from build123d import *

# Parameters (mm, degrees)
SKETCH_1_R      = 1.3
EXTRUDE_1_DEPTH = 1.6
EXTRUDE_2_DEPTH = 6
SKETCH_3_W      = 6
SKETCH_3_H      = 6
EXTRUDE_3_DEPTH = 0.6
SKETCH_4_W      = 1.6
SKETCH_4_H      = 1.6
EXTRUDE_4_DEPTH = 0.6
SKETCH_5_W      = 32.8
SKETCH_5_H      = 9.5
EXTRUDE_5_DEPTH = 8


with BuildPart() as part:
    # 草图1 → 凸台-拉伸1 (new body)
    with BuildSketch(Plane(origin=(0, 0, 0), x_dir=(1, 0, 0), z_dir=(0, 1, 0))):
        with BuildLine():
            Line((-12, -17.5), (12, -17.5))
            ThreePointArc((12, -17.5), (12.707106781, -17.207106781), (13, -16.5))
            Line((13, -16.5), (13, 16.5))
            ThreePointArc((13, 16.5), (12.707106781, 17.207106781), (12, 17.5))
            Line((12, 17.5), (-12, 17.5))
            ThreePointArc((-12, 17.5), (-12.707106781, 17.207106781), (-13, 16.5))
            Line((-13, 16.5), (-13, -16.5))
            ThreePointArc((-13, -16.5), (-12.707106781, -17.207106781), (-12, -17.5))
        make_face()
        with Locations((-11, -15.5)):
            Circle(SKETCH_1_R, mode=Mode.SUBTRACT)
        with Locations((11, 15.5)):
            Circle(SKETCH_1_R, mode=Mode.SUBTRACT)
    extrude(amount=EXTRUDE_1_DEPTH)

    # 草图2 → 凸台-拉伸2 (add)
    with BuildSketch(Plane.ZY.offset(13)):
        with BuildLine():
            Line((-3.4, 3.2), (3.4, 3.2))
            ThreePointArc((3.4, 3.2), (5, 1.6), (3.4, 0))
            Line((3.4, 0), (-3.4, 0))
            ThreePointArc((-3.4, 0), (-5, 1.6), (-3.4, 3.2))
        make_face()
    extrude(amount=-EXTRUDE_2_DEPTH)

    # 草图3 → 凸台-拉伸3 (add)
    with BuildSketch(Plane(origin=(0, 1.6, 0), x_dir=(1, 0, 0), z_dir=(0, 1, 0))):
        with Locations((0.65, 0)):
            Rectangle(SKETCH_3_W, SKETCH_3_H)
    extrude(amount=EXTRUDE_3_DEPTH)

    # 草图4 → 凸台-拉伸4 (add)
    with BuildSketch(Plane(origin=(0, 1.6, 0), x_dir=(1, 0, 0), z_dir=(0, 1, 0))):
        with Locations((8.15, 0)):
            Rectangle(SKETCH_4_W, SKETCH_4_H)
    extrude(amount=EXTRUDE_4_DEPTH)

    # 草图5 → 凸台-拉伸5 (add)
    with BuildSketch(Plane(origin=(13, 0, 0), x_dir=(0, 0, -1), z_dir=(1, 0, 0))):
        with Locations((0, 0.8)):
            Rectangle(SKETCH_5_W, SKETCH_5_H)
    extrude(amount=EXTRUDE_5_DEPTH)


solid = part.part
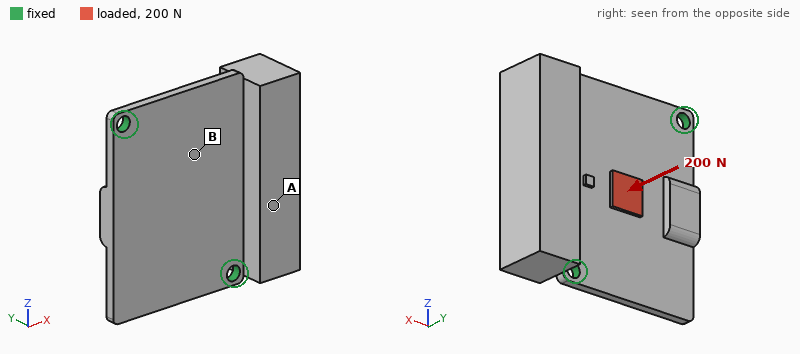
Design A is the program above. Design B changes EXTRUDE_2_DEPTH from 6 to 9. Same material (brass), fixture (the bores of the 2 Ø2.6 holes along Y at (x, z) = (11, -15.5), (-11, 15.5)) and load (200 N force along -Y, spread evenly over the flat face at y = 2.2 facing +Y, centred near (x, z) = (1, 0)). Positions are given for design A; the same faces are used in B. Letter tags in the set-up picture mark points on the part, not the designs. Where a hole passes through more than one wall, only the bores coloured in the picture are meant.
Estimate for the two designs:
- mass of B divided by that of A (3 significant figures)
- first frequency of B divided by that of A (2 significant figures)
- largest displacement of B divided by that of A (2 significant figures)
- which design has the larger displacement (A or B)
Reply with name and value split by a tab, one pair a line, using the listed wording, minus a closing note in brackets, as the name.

mass of B divided by that of A	1.01
first frequency of B divided by that of A	1.0
largest displacement of B divided by that of A	0.89
which design has the larger displacement	A
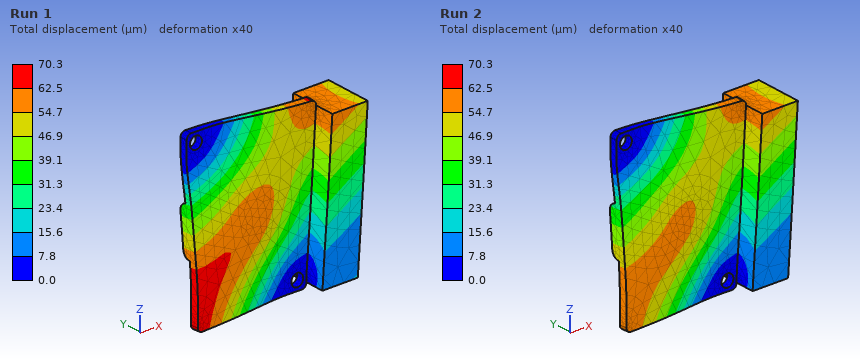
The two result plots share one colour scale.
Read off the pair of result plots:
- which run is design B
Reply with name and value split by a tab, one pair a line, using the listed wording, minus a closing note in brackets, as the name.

which run is design B	Run 2
